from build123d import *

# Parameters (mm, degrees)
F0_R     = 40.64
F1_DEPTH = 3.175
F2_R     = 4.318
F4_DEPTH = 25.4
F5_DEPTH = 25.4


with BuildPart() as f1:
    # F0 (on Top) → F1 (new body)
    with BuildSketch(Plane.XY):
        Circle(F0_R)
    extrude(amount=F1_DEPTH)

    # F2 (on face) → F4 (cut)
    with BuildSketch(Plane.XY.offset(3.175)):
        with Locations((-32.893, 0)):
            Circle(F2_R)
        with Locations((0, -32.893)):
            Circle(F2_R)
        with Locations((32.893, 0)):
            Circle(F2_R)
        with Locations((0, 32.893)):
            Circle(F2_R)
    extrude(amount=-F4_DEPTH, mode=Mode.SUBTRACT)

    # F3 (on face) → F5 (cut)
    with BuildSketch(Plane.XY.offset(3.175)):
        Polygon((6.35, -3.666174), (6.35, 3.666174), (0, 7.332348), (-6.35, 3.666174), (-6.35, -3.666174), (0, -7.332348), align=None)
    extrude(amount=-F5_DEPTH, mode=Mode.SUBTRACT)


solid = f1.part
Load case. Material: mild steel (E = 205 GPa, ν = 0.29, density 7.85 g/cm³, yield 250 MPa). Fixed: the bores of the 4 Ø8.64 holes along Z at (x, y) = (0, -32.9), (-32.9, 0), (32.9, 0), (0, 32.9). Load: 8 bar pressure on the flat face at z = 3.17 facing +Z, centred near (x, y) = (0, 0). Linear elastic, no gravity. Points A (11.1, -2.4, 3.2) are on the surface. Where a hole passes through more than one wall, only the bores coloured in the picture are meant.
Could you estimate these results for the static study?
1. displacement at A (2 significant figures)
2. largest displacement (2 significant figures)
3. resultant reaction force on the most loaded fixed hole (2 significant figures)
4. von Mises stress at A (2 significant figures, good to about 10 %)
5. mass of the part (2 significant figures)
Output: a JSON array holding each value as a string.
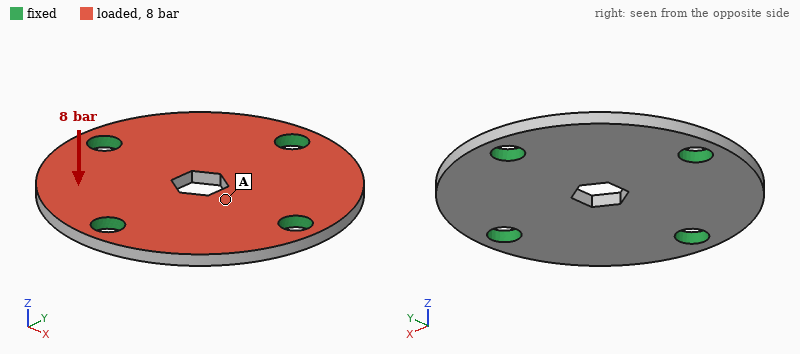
["20 µm", "24 µm", "960 N", "21 MPa", "120 g"]
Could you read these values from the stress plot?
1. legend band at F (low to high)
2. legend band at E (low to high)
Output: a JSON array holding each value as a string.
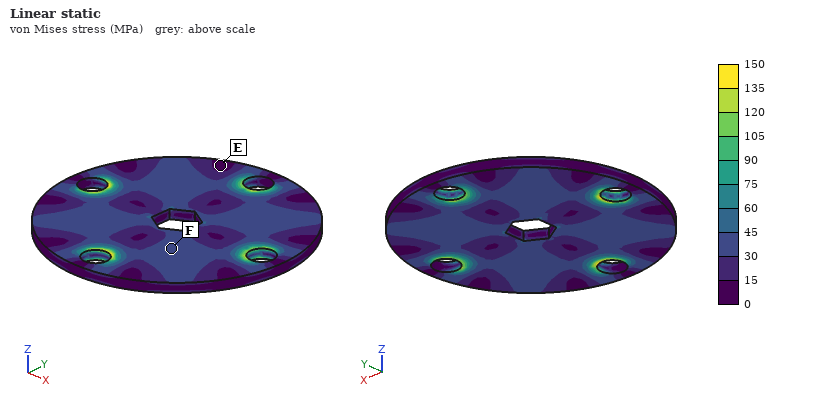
["30 to 45 MPa", "0 to 15 MPa"]
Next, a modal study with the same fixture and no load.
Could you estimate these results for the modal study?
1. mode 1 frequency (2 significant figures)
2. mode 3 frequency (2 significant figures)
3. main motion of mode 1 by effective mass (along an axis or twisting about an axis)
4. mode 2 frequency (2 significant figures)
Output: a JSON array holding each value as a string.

["7000 Hz", "7600 Hz", "along Z", "7400 Hz"]
